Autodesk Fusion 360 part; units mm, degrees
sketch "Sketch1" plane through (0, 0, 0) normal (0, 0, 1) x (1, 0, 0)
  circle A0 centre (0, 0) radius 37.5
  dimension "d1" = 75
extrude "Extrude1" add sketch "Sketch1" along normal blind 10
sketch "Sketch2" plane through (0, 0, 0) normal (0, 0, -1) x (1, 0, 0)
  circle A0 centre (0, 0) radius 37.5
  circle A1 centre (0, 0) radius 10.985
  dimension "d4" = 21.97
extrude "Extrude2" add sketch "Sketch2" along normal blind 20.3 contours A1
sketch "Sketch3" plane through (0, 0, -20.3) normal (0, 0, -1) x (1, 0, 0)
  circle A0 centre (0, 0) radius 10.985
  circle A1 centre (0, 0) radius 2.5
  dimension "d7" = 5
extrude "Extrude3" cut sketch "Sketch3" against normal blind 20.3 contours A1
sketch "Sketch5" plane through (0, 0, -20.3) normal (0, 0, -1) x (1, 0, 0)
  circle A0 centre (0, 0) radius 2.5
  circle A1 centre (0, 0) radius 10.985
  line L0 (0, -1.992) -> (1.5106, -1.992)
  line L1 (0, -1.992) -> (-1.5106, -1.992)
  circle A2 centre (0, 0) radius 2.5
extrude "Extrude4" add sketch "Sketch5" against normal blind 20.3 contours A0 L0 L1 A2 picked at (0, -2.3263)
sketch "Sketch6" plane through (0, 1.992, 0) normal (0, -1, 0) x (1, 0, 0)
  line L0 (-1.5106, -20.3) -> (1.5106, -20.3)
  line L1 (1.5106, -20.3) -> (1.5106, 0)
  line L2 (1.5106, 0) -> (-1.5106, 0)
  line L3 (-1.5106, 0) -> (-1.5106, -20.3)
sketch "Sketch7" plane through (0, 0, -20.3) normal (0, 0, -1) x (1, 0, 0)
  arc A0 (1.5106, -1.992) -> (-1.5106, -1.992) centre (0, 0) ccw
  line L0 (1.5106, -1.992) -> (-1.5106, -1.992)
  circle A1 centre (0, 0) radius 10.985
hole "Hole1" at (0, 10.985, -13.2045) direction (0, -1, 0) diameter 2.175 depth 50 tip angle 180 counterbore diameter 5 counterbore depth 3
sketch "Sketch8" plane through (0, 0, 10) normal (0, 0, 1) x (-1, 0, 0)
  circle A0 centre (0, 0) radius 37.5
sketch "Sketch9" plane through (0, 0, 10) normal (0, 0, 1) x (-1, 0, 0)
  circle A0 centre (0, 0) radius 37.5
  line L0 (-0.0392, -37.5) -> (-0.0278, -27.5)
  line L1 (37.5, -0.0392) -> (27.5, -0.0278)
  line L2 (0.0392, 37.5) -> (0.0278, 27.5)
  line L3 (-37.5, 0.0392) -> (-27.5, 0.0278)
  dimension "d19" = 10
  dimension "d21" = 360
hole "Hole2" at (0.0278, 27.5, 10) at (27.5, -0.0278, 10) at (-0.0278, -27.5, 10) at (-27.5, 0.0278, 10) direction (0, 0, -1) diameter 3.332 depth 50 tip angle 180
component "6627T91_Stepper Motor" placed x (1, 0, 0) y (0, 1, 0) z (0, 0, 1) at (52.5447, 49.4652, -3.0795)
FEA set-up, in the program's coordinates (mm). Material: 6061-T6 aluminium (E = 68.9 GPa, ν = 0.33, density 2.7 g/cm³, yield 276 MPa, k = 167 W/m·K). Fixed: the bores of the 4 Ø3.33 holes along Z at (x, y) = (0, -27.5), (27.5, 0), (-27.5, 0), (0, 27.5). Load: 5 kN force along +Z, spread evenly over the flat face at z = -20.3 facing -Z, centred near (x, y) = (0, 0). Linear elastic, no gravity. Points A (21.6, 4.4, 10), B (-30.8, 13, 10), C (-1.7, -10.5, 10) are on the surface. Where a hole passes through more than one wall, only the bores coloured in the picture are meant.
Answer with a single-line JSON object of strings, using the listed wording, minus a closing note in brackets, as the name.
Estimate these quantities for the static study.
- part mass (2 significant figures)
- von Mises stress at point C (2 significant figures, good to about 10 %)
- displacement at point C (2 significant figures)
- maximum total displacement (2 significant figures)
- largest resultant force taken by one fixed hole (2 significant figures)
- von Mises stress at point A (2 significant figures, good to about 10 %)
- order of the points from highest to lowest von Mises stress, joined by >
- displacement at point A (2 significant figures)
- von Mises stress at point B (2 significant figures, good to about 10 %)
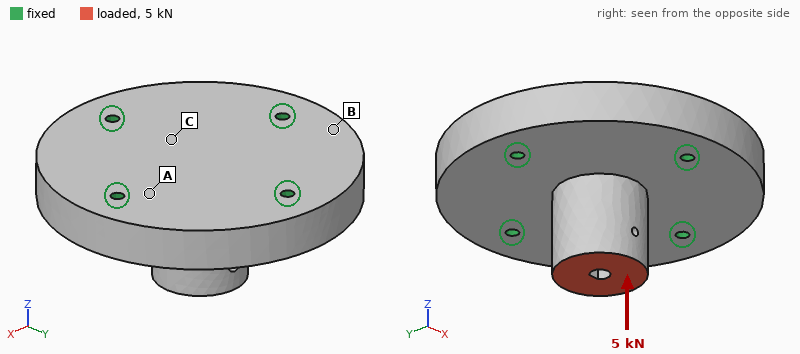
{"part mass": "140 g", "von Mises stress at point C": "20 MPa", "displacement at point C": "12 µm", "maximum total displacement": "18 µm", "largest resultant force taken by one fixed hole": "1.3 kN", "von Mises stress at point A": "9.5 MPa", "order of the points from highest to lowest von Mises stress, joined by >": "C > A > B", "displacement at point A": "4.8 µm", "von Mises stress at point B": "4.9 MPa"}
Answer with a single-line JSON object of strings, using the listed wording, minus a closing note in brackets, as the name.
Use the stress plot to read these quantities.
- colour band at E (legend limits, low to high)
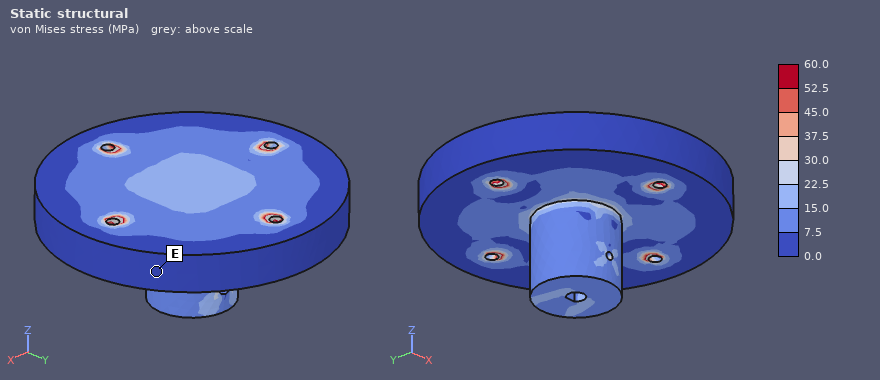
{"colour band at E": "0.0 to 7.5 MPa"}
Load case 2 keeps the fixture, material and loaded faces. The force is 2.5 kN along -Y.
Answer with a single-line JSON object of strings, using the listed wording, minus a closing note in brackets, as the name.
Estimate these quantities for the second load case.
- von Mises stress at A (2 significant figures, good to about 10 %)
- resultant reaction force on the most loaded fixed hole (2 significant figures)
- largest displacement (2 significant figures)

{"von Mises stress at A": "6.3 MPa", "resultant reaction force on the most loaded fixed hole": "1.5 kN", "largest displacement": "40 µm"}
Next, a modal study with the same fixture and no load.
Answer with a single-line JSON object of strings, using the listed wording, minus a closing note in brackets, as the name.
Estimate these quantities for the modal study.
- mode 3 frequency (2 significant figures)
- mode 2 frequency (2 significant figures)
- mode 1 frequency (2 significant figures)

{"mode 3 frequency": "14 kHz", "mode 2 frequency": "14 kHz", "mode 1 frequency": "14 kHz"}
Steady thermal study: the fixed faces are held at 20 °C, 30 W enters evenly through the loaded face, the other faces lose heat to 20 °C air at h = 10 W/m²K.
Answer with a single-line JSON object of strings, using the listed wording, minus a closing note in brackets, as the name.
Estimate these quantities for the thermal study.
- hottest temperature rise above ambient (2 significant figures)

{"hottest temperature rise above ambient": "16 K"}
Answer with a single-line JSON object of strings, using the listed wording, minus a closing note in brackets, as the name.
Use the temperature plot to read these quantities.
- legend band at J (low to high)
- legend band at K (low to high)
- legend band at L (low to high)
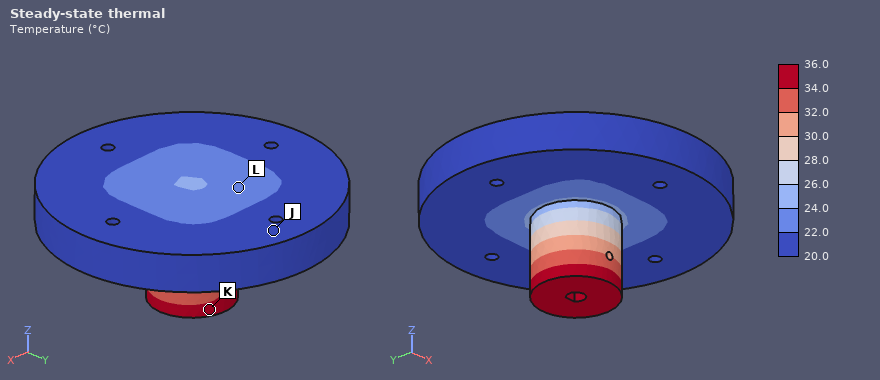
{"legend band at J": "20.0 to 22.0 °C", "legend band at K": "34.0 to 36.0 °C", "legend band at L": "22.0 to 24.0 °C"}
